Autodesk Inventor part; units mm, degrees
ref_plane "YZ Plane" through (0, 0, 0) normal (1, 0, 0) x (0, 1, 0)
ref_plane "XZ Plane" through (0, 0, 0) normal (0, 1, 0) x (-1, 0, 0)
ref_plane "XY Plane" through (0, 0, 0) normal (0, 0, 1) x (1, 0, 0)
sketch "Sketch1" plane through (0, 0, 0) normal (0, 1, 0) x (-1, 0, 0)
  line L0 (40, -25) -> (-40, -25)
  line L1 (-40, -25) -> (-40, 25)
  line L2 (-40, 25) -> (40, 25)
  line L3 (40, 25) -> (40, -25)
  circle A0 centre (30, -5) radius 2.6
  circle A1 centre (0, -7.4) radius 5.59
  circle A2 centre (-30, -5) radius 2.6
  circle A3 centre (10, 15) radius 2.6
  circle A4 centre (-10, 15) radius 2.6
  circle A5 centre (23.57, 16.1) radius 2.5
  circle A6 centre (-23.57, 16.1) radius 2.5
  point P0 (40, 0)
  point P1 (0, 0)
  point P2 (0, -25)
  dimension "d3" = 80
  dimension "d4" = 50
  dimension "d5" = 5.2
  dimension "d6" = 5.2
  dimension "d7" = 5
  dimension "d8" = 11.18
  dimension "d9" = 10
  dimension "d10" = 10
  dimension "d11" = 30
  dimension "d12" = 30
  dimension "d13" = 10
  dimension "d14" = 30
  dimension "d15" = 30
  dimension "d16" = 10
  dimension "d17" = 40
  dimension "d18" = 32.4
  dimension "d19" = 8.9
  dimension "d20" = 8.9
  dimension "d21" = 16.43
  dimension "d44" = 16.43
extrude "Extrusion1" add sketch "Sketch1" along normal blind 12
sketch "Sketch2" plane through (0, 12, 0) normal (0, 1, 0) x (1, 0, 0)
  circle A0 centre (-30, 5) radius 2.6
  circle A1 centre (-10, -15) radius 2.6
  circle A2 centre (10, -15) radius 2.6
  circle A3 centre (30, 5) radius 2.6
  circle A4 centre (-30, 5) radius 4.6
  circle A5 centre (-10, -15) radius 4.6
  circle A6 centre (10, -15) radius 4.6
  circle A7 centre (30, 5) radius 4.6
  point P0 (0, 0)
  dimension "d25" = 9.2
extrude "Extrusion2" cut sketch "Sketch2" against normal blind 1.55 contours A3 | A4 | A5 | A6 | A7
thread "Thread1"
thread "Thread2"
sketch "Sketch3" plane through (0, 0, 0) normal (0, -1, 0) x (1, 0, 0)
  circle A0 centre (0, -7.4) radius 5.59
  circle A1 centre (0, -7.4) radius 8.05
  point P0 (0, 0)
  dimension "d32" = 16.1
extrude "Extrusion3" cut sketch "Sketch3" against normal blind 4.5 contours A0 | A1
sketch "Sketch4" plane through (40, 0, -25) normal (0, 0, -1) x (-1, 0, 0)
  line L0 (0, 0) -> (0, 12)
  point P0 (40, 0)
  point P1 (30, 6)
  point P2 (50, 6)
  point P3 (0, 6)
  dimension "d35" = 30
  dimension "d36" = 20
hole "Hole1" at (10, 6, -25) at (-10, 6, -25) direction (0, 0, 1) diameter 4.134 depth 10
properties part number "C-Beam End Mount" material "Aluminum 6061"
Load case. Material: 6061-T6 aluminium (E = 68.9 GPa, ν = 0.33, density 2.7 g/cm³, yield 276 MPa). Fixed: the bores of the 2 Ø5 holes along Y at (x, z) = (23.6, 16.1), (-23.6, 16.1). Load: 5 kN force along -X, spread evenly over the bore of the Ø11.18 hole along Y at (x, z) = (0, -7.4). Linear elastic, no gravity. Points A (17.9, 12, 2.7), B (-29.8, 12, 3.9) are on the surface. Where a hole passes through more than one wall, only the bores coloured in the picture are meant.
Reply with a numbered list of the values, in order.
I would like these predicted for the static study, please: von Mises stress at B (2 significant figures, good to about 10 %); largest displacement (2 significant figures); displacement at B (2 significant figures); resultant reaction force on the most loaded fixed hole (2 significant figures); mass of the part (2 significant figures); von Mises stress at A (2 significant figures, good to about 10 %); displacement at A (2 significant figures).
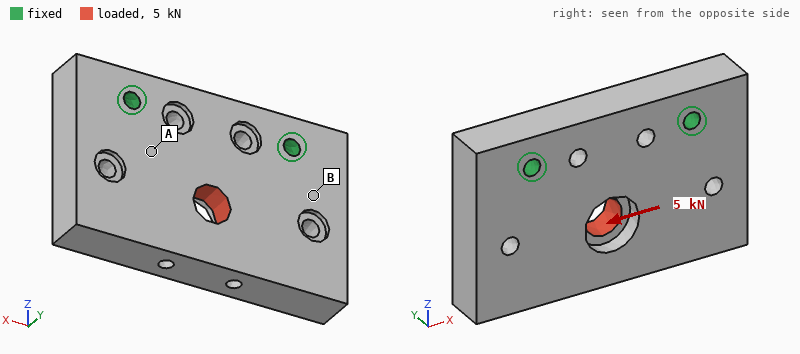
1. 5.6 MPa
2. 16 µm
3. 5.9 µm
4. 3.4 kN
5. 120 g
6. 15 MPa
7. 5.8 µm
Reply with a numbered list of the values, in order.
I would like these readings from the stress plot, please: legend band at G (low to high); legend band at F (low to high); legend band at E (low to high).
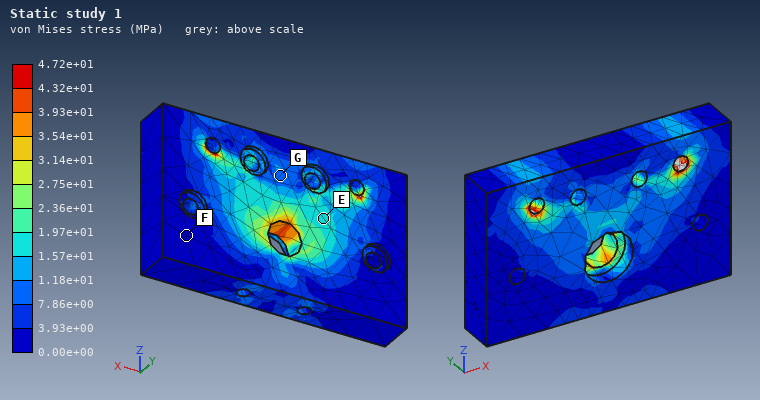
1. 7.86e+00 to 1.18e+01 MPa
2. 0.00e+00 to 3.93e+00 MPa
3. 1.57e+01 to 1.97e+01 MPa
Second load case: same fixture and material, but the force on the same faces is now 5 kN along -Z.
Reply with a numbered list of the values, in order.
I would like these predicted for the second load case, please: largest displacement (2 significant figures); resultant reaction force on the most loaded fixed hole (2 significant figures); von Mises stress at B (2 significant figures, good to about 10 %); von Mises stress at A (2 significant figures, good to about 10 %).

1. 20 µm
2. 2.7 kN
3. 6.8 MPa
4. 17 MPa
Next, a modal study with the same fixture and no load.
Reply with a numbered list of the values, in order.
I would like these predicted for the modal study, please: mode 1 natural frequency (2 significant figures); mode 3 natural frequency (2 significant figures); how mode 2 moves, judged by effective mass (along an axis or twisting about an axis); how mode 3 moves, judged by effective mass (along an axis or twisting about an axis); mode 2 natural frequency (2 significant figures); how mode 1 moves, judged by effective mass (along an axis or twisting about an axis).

1. 4400 Hz
2. 11 kHz
3. twisting about Z
4. along X
5. 6800 Hz
6. along Y
